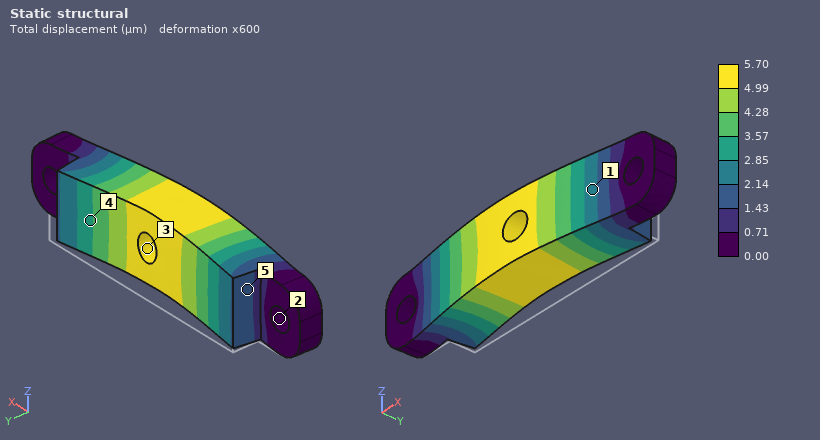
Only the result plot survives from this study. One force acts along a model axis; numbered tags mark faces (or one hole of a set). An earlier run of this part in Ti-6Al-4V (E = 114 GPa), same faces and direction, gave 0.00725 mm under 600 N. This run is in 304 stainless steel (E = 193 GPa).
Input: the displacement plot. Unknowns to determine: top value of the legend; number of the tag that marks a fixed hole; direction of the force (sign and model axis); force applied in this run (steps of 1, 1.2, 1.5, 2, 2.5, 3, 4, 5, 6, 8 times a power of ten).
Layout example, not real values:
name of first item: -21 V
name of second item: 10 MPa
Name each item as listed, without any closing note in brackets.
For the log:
top value of the legend: 5.70 µm
number of the tag that marks a fixed hole: 2
direction of the force: -Y
force applied in this run: 800 N
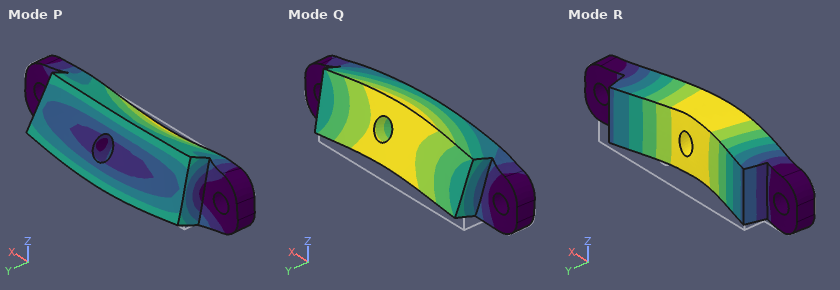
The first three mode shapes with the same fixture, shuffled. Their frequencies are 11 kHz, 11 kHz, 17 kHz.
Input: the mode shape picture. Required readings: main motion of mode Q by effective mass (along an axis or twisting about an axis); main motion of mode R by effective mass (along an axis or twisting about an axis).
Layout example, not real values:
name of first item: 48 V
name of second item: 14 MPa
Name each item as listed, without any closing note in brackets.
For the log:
main motion of mode Q by effective mass: along Z
main motion of mode R by effective mass: along Y
